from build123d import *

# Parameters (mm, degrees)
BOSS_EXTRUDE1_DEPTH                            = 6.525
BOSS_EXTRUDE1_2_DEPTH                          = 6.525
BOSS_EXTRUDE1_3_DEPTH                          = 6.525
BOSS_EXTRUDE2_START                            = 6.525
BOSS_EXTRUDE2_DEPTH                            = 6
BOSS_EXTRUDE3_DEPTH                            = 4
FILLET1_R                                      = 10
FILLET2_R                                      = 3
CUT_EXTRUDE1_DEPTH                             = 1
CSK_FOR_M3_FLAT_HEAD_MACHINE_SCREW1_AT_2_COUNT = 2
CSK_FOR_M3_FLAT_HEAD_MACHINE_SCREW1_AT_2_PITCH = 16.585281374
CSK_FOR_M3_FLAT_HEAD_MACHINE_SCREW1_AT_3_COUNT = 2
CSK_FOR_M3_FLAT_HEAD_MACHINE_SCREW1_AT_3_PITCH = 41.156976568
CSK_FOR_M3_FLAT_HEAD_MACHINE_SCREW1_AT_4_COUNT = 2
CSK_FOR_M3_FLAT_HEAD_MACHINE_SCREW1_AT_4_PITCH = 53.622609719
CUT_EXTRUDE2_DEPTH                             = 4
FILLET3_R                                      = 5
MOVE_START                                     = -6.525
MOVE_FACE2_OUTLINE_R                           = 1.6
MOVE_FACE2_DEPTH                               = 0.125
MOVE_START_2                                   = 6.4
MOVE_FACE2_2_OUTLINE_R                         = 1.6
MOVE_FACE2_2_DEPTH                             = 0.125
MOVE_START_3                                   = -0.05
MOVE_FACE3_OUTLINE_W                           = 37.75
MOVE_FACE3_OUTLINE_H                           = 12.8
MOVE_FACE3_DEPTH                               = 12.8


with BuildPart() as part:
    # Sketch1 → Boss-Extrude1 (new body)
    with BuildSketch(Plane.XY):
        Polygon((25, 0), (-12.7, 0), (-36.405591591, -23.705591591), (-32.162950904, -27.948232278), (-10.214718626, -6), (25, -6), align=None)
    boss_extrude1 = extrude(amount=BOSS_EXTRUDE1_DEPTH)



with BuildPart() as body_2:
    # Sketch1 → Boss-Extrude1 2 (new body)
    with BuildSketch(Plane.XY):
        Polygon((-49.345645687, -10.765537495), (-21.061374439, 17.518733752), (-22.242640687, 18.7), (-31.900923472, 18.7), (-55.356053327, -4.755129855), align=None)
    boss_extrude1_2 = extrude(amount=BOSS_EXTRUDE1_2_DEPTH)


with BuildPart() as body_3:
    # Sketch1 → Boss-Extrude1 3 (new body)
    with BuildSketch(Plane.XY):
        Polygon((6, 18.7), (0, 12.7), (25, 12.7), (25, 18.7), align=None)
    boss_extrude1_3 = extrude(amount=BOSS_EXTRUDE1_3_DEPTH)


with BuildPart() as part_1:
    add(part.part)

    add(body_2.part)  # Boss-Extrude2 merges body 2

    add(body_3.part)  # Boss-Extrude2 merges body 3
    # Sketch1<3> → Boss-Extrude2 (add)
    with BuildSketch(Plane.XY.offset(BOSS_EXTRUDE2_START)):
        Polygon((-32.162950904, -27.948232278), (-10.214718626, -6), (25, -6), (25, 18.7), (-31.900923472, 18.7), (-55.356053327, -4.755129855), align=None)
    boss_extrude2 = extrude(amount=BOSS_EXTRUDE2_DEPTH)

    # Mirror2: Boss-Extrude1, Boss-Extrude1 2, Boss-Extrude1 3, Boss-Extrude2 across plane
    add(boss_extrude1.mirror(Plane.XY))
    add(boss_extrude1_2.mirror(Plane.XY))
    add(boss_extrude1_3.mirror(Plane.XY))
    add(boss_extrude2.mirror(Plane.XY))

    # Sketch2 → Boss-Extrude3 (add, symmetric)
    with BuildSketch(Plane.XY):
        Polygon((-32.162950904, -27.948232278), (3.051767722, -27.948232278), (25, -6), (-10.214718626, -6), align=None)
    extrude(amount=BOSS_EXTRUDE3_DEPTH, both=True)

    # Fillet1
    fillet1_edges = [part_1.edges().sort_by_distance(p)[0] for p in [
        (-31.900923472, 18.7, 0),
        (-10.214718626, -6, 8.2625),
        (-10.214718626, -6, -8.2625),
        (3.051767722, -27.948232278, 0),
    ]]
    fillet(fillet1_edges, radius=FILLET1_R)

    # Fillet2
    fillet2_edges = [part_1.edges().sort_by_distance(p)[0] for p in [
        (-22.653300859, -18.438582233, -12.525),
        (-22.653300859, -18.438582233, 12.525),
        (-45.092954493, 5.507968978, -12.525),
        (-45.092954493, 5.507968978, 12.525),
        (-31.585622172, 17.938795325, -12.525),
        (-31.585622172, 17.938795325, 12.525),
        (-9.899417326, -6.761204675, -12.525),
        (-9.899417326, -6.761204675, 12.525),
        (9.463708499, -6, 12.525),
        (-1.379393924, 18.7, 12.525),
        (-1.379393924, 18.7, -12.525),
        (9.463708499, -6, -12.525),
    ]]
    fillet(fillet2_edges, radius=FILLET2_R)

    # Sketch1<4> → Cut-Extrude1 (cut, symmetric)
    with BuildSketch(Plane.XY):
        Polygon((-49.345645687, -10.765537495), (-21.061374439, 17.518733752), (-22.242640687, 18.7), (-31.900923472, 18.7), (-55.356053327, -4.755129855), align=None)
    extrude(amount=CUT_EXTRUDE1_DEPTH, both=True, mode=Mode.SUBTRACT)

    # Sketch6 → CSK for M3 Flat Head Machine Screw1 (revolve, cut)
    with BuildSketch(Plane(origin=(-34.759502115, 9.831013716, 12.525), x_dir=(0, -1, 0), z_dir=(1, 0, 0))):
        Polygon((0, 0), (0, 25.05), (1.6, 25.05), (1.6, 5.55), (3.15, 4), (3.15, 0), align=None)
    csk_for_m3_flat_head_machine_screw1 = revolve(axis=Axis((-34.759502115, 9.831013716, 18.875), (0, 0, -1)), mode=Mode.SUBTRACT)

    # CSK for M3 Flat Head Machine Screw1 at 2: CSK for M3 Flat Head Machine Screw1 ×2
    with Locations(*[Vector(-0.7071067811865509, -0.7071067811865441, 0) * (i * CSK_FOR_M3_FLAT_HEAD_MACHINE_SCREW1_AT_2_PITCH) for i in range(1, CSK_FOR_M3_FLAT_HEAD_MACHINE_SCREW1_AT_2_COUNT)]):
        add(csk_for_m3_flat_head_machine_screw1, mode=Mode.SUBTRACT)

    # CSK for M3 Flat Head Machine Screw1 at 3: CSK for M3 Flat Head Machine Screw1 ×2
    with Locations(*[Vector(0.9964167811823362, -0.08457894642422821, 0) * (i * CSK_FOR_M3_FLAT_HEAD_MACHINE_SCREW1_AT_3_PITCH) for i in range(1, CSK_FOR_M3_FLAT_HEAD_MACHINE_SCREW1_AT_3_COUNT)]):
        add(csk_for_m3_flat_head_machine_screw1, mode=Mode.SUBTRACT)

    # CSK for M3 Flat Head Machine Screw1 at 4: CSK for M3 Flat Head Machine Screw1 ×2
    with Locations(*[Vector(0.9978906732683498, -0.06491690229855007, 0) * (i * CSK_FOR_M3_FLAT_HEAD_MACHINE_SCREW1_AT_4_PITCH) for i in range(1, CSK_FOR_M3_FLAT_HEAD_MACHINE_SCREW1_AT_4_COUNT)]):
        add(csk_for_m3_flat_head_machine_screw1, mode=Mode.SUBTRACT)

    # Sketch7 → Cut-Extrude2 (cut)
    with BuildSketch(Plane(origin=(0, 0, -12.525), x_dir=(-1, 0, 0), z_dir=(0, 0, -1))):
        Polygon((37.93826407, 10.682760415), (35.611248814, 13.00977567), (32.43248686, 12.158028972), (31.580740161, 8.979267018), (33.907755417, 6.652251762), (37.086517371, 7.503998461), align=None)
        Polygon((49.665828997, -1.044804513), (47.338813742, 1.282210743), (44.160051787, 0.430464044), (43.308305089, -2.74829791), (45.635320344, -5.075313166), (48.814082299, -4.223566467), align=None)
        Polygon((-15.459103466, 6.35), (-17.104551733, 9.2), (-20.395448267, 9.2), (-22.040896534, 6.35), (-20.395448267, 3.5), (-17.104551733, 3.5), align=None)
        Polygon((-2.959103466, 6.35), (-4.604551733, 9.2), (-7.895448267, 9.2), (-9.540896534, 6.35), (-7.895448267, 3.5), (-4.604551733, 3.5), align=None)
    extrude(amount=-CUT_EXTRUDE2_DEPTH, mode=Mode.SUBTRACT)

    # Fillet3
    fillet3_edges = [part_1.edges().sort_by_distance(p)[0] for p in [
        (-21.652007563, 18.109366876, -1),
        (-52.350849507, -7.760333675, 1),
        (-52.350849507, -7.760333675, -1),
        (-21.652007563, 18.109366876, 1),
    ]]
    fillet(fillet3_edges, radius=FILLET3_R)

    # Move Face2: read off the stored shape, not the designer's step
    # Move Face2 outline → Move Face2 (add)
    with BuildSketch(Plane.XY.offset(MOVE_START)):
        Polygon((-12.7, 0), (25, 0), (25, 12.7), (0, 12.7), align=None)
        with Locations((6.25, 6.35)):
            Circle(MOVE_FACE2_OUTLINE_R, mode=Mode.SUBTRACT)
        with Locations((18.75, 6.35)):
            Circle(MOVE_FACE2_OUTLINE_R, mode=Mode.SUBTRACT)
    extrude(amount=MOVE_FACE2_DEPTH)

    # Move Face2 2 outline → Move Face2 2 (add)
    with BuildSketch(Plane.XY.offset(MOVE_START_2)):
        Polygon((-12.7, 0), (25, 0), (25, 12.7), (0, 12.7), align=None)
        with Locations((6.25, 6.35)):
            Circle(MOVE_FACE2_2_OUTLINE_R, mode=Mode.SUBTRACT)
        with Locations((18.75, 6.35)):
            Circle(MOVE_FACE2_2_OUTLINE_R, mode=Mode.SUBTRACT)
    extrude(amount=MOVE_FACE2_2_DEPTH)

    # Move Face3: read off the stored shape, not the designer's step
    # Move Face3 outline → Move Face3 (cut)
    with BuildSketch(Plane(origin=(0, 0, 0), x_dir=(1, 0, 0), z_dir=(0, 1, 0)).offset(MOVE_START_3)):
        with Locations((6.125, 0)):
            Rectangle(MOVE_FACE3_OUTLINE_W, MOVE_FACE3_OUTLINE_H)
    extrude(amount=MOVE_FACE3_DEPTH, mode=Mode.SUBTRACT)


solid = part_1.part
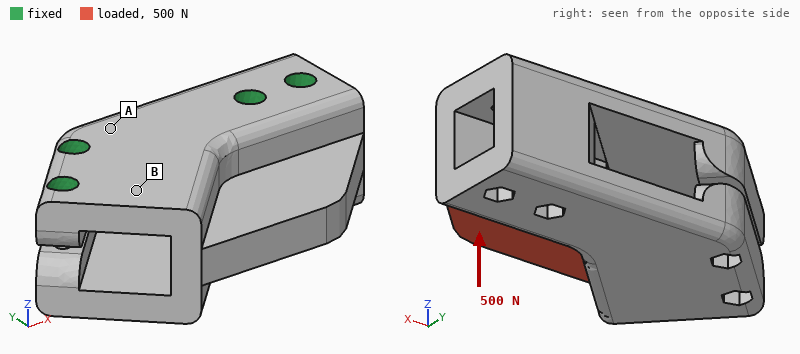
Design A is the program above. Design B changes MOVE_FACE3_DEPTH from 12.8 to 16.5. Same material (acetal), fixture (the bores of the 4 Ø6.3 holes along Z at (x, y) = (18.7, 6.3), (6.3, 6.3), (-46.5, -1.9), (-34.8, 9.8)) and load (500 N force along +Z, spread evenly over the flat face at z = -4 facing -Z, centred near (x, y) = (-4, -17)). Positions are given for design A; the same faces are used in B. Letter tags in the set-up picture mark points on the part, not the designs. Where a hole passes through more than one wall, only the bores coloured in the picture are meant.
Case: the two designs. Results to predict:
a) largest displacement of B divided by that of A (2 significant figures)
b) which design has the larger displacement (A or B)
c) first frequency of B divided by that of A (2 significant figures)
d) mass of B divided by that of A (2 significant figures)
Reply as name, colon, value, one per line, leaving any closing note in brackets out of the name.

largest displacement of B divided by that of A: 1.1
which design has the larger displacement: B
first frequency of B divided by that of A: 0.93
mass of B divided by that of A: 0.97
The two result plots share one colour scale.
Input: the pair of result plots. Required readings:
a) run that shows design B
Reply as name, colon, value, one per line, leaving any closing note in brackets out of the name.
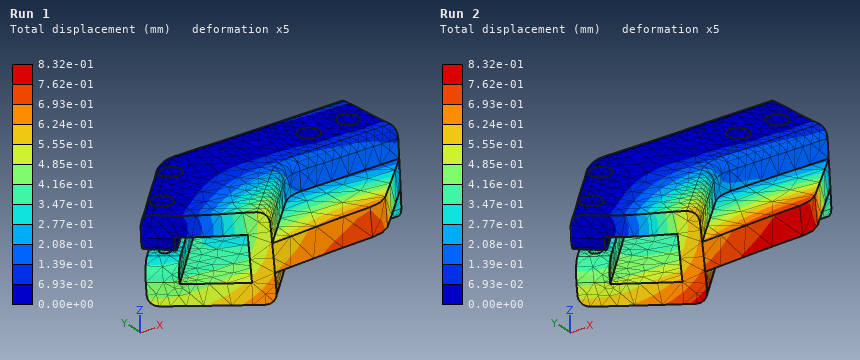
run that shows design B: Run 2
